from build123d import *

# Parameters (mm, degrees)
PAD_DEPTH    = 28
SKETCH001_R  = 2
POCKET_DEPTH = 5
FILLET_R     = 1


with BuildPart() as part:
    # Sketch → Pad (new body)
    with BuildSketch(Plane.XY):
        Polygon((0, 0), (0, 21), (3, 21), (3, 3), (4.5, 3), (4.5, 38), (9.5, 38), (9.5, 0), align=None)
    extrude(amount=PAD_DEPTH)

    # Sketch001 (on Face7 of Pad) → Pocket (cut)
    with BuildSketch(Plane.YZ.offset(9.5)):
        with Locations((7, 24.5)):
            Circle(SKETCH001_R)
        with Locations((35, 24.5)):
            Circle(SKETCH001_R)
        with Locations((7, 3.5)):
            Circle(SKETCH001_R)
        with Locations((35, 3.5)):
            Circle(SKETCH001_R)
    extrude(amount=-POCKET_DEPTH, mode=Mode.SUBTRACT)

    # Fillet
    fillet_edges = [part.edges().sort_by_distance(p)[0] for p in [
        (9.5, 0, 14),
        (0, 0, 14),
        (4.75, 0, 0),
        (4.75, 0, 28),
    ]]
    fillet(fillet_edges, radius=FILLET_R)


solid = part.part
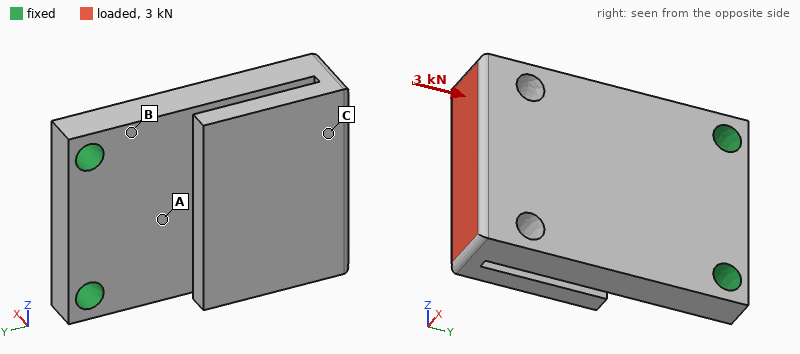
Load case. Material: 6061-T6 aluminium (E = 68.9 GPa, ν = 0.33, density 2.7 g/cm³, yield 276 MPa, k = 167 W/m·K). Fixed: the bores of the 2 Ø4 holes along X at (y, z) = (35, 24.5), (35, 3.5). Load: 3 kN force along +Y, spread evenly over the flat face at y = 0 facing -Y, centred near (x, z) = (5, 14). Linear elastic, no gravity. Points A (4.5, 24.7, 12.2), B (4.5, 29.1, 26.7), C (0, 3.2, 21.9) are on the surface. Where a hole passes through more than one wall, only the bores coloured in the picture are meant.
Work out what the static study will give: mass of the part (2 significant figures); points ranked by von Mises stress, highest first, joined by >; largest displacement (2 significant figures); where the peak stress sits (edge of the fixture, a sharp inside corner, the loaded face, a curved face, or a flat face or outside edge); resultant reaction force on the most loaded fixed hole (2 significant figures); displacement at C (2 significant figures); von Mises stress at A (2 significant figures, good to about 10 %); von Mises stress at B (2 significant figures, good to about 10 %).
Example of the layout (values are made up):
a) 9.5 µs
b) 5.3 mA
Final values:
a) 19 g
b) B > A > C
c) 0.24 mm
d) a curved face
e) 1.5 kN
f) 0.20 mm
g) 68 MPa
h) 93 MPa
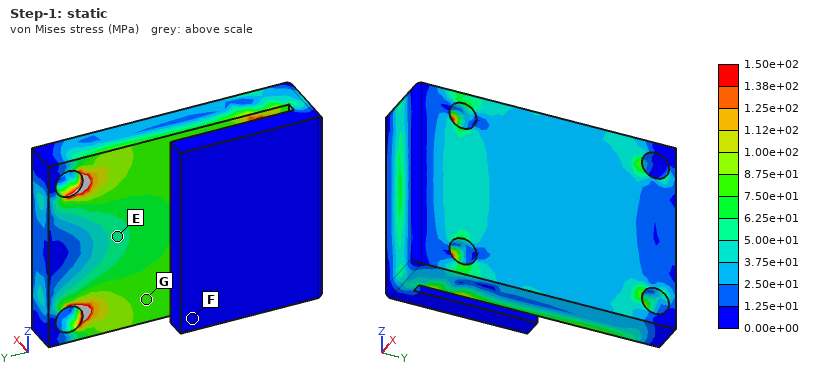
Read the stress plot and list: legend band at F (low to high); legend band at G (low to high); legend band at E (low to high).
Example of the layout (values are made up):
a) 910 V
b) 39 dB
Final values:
a) 0.00e+00 to 1.25e+01 MPa
b) 7.50e+01 to 8.75e+01 MPa
c) 5.00e+01 to 6.25e+01 MPa
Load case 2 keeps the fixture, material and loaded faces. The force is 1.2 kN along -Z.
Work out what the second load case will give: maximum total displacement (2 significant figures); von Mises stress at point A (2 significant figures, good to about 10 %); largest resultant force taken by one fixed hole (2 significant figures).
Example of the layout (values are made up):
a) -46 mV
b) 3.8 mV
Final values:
a) 67 µm
b) 37 MPa
c) 2.0 kN
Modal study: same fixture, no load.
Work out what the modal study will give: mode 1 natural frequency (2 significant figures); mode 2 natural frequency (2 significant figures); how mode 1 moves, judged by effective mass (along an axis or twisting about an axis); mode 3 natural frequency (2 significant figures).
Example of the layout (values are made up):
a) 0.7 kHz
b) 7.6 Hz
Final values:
a) 2500 Hz
b) 4700 Hz
c) along X
d) 5500 Hz
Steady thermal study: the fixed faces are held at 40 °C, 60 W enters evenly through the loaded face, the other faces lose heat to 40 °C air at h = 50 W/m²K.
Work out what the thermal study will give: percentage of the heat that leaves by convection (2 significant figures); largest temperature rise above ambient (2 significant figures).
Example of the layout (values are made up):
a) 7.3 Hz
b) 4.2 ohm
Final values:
a) 17 %
b) 86 K
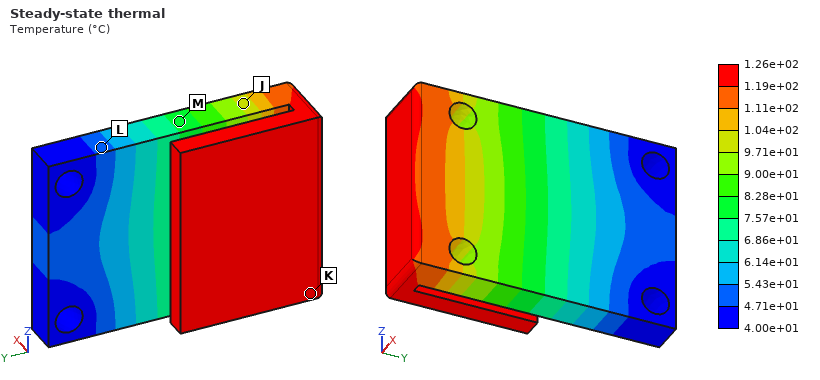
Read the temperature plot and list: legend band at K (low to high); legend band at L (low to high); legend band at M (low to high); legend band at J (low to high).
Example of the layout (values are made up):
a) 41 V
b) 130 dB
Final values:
a) 1.19e+02 to 1.26e+02 °C
b) 4.71e+01 to 5.43e+01 °C
c) 7.57e+01 to 8.28e+01 °C
d) 9.71e+01 to 1.04e+02 °C
